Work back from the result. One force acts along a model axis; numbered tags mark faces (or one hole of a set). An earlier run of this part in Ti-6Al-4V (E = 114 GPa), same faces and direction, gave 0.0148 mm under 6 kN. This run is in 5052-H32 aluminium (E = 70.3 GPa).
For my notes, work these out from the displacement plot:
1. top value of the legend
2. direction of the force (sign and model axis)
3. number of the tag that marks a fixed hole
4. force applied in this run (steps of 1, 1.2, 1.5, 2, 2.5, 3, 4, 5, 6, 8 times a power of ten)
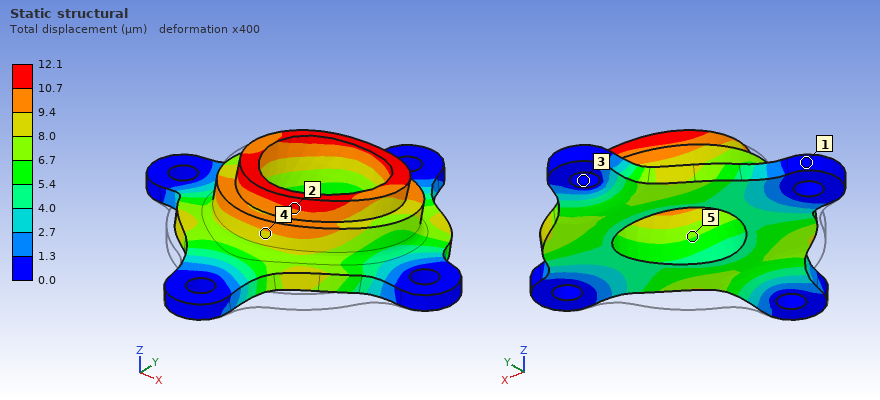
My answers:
12.1 µm
+Y
3
3 kN
